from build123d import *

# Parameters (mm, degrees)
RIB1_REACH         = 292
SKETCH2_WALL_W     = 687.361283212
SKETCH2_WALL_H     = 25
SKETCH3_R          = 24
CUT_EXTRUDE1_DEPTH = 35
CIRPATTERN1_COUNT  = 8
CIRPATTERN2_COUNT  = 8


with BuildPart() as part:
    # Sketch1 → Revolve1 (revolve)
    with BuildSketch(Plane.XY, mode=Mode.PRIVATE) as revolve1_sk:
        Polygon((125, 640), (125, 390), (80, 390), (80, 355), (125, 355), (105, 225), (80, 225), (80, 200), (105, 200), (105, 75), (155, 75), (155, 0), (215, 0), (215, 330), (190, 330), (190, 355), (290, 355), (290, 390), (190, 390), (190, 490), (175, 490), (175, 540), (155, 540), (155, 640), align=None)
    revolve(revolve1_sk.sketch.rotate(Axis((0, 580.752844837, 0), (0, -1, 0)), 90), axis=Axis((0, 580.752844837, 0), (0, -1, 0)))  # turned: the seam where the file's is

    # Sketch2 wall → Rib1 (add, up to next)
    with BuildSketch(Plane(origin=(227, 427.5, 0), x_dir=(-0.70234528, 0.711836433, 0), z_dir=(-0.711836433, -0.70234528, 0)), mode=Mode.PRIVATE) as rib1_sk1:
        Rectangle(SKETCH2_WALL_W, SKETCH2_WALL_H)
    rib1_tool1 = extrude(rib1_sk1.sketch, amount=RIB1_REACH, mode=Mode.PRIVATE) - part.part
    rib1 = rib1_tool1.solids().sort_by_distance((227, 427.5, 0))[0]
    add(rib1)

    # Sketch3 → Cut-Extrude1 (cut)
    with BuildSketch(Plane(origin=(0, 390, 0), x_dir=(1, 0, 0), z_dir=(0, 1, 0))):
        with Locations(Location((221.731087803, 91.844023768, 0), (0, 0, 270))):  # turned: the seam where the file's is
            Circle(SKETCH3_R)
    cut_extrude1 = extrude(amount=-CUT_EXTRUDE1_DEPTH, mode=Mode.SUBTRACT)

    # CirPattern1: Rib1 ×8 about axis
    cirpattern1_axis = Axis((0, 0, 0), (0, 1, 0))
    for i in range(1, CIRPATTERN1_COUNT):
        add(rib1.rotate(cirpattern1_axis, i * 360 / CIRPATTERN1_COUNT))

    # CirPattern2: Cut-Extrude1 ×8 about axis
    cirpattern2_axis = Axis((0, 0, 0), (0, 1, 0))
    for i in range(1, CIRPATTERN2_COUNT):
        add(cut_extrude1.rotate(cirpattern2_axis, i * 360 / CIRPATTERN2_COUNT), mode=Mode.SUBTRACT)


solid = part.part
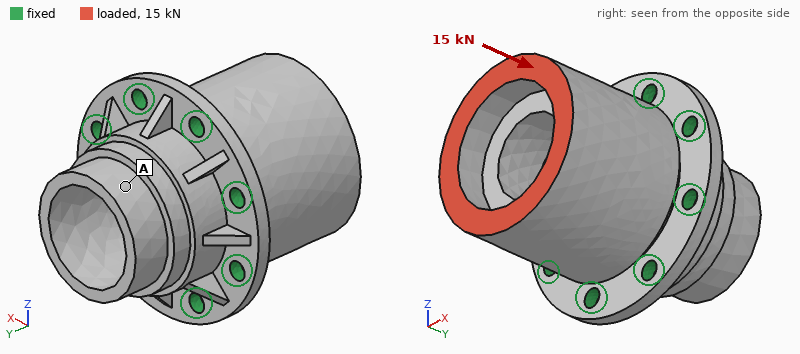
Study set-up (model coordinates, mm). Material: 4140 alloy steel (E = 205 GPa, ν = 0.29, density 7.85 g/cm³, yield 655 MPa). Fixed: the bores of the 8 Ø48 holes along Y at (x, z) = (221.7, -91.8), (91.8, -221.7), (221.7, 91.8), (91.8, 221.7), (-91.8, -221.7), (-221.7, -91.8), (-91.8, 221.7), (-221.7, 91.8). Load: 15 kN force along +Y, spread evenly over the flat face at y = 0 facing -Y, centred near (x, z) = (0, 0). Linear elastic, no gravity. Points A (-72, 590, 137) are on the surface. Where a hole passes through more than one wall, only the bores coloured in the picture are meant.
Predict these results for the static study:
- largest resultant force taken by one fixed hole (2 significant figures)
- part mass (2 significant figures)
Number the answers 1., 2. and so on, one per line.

1. 1.9 kN
2. 430 kg
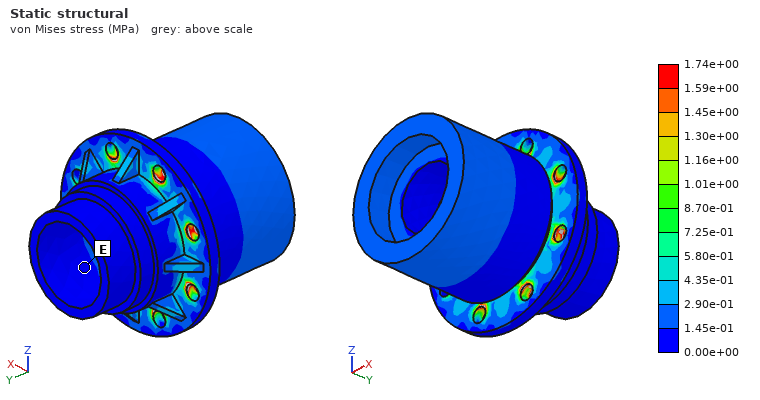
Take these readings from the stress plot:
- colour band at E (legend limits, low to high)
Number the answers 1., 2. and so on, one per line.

1. 0.00e+00 to 1.45e-01 MPa
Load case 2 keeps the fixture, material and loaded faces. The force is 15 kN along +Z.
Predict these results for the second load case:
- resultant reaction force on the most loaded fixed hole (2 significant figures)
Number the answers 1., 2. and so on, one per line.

1. 6.3 kN
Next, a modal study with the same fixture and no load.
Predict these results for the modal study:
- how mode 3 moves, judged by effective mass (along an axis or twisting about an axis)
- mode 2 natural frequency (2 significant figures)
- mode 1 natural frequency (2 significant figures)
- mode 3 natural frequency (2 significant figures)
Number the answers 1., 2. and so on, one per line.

1. along Y
2. 820 Hz
3. 820 Hz
4. 1400 Hz
